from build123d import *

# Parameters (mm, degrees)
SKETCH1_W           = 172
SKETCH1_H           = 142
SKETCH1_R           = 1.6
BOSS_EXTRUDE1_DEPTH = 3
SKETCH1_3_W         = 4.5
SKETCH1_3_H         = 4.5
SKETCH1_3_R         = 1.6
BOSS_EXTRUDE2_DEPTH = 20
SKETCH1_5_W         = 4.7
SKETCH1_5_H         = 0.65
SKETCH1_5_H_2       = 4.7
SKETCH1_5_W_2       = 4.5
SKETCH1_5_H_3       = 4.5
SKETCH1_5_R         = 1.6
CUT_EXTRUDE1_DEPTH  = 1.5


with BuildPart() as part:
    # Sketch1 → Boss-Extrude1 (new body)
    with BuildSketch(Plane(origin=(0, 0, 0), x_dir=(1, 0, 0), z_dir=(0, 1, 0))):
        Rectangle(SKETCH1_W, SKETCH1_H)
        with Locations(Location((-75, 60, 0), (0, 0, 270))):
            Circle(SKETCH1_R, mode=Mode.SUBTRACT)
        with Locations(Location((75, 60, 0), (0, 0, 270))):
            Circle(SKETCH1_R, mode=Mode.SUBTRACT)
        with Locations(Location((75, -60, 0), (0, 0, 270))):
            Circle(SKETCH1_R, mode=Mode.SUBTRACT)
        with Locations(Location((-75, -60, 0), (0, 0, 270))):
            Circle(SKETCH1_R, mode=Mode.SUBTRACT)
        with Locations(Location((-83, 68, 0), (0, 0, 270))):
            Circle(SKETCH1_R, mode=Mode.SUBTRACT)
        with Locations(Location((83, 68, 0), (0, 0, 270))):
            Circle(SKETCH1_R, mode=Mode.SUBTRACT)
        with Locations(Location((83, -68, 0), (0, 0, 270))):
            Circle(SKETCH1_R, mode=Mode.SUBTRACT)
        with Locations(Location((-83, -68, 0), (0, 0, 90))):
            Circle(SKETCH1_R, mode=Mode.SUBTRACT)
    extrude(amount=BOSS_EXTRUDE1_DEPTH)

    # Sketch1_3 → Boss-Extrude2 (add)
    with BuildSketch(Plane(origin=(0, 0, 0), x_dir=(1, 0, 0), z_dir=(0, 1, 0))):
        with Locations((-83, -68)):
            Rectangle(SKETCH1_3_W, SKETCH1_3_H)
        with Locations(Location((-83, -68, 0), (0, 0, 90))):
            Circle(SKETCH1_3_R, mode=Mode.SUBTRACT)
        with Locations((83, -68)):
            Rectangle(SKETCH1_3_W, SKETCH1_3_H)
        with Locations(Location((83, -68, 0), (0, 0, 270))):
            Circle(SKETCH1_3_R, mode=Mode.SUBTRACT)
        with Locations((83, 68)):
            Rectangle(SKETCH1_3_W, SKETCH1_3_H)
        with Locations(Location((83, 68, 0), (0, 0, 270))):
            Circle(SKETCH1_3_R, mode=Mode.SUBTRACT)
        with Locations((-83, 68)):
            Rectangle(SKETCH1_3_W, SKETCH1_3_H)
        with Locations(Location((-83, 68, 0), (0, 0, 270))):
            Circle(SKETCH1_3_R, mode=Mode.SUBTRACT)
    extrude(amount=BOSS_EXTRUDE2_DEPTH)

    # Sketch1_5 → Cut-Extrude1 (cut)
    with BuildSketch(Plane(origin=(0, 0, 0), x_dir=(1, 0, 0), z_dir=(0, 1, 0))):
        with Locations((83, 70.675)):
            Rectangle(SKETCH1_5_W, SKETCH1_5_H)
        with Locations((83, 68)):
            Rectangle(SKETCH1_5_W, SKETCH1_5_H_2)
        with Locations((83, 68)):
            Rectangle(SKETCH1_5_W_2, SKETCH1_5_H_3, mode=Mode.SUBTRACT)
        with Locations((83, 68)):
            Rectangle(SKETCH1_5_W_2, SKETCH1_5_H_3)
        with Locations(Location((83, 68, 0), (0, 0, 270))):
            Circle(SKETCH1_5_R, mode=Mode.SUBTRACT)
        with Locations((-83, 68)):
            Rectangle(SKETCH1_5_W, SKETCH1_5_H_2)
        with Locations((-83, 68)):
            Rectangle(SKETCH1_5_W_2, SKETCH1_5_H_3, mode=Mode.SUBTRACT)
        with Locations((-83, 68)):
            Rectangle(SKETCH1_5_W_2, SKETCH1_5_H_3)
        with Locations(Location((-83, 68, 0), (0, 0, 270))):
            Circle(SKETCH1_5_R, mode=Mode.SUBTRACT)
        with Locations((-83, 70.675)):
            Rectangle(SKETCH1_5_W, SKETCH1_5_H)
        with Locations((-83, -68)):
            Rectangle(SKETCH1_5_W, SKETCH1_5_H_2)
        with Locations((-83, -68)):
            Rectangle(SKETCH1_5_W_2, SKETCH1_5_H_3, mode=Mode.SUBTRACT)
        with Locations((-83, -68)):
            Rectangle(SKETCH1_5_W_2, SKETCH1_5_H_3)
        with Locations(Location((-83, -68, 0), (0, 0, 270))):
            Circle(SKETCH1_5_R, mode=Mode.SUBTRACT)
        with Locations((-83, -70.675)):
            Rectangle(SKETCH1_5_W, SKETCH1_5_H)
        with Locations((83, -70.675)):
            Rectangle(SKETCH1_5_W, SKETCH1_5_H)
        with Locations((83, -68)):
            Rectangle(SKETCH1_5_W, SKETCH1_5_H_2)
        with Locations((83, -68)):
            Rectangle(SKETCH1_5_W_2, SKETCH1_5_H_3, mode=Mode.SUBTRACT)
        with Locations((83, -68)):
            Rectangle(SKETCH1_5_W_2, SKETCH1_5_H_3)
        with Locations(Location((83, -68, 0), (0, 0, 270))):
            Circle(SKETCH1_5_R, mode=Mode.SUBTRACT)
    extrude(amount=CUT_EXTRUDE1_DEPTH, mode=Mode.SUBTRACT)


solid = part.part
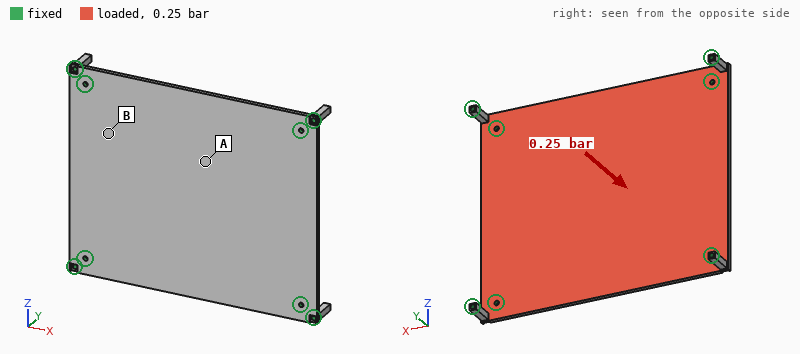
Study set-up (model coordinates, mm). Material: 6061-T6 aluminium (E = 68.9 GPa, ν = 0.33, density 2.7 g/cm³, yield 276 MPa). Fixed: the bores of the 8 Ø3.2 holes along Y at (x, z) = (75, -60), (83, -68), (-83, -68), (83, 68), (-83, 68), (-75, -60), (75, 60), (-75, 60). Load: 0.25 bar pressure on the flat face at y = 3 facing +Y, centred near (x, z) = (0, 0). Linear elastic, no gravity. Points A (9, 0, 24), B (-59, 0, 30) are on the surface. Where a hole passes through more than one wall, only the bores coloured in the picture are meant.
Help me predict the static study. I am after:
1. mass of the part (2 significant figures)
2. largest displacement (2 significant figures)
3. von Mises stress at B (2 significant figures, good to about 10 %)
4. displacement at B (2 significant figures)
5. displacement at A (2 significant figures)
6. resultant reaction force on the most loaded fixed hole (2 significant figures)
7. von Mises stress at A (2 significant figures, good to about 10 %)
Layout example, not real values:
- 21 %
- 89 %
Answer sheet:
- 200 g
- 0.43 mm
- 8.5 MPa
- 0.17 mm
- 0.41 mm
- 260 N
- 18 MPa
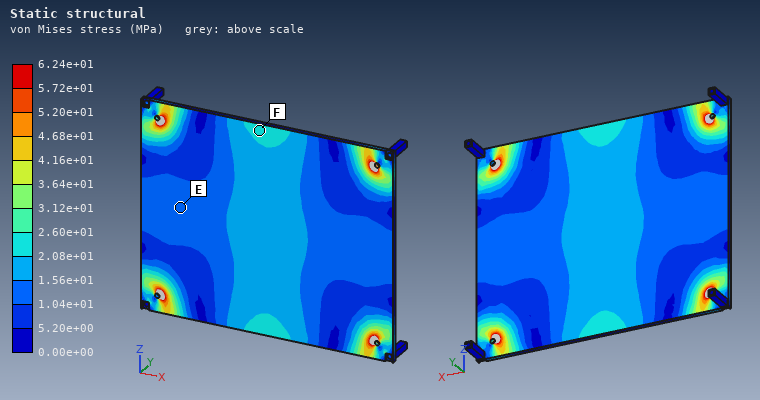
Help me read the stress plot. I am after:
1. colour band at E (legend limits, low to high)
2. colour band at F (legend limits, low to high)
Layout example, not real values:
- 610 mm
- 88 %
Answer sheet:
- 1.04e+01 to 1.56e+01 MPa
- 2.08e+01 to 2.60e+01 MPa
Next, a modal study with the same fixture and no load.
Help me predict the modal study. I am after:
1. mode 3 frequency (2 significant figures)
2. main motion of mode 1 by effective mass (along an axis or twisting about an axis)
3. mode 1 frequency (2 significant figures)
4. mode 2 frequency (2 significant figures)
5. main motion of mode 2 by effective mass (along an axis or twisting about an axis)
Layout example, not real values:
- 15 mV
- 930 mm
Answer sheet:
- 1000 Hz
- along Y
- 510 Hz
- 810 Hz
- twisting about X
